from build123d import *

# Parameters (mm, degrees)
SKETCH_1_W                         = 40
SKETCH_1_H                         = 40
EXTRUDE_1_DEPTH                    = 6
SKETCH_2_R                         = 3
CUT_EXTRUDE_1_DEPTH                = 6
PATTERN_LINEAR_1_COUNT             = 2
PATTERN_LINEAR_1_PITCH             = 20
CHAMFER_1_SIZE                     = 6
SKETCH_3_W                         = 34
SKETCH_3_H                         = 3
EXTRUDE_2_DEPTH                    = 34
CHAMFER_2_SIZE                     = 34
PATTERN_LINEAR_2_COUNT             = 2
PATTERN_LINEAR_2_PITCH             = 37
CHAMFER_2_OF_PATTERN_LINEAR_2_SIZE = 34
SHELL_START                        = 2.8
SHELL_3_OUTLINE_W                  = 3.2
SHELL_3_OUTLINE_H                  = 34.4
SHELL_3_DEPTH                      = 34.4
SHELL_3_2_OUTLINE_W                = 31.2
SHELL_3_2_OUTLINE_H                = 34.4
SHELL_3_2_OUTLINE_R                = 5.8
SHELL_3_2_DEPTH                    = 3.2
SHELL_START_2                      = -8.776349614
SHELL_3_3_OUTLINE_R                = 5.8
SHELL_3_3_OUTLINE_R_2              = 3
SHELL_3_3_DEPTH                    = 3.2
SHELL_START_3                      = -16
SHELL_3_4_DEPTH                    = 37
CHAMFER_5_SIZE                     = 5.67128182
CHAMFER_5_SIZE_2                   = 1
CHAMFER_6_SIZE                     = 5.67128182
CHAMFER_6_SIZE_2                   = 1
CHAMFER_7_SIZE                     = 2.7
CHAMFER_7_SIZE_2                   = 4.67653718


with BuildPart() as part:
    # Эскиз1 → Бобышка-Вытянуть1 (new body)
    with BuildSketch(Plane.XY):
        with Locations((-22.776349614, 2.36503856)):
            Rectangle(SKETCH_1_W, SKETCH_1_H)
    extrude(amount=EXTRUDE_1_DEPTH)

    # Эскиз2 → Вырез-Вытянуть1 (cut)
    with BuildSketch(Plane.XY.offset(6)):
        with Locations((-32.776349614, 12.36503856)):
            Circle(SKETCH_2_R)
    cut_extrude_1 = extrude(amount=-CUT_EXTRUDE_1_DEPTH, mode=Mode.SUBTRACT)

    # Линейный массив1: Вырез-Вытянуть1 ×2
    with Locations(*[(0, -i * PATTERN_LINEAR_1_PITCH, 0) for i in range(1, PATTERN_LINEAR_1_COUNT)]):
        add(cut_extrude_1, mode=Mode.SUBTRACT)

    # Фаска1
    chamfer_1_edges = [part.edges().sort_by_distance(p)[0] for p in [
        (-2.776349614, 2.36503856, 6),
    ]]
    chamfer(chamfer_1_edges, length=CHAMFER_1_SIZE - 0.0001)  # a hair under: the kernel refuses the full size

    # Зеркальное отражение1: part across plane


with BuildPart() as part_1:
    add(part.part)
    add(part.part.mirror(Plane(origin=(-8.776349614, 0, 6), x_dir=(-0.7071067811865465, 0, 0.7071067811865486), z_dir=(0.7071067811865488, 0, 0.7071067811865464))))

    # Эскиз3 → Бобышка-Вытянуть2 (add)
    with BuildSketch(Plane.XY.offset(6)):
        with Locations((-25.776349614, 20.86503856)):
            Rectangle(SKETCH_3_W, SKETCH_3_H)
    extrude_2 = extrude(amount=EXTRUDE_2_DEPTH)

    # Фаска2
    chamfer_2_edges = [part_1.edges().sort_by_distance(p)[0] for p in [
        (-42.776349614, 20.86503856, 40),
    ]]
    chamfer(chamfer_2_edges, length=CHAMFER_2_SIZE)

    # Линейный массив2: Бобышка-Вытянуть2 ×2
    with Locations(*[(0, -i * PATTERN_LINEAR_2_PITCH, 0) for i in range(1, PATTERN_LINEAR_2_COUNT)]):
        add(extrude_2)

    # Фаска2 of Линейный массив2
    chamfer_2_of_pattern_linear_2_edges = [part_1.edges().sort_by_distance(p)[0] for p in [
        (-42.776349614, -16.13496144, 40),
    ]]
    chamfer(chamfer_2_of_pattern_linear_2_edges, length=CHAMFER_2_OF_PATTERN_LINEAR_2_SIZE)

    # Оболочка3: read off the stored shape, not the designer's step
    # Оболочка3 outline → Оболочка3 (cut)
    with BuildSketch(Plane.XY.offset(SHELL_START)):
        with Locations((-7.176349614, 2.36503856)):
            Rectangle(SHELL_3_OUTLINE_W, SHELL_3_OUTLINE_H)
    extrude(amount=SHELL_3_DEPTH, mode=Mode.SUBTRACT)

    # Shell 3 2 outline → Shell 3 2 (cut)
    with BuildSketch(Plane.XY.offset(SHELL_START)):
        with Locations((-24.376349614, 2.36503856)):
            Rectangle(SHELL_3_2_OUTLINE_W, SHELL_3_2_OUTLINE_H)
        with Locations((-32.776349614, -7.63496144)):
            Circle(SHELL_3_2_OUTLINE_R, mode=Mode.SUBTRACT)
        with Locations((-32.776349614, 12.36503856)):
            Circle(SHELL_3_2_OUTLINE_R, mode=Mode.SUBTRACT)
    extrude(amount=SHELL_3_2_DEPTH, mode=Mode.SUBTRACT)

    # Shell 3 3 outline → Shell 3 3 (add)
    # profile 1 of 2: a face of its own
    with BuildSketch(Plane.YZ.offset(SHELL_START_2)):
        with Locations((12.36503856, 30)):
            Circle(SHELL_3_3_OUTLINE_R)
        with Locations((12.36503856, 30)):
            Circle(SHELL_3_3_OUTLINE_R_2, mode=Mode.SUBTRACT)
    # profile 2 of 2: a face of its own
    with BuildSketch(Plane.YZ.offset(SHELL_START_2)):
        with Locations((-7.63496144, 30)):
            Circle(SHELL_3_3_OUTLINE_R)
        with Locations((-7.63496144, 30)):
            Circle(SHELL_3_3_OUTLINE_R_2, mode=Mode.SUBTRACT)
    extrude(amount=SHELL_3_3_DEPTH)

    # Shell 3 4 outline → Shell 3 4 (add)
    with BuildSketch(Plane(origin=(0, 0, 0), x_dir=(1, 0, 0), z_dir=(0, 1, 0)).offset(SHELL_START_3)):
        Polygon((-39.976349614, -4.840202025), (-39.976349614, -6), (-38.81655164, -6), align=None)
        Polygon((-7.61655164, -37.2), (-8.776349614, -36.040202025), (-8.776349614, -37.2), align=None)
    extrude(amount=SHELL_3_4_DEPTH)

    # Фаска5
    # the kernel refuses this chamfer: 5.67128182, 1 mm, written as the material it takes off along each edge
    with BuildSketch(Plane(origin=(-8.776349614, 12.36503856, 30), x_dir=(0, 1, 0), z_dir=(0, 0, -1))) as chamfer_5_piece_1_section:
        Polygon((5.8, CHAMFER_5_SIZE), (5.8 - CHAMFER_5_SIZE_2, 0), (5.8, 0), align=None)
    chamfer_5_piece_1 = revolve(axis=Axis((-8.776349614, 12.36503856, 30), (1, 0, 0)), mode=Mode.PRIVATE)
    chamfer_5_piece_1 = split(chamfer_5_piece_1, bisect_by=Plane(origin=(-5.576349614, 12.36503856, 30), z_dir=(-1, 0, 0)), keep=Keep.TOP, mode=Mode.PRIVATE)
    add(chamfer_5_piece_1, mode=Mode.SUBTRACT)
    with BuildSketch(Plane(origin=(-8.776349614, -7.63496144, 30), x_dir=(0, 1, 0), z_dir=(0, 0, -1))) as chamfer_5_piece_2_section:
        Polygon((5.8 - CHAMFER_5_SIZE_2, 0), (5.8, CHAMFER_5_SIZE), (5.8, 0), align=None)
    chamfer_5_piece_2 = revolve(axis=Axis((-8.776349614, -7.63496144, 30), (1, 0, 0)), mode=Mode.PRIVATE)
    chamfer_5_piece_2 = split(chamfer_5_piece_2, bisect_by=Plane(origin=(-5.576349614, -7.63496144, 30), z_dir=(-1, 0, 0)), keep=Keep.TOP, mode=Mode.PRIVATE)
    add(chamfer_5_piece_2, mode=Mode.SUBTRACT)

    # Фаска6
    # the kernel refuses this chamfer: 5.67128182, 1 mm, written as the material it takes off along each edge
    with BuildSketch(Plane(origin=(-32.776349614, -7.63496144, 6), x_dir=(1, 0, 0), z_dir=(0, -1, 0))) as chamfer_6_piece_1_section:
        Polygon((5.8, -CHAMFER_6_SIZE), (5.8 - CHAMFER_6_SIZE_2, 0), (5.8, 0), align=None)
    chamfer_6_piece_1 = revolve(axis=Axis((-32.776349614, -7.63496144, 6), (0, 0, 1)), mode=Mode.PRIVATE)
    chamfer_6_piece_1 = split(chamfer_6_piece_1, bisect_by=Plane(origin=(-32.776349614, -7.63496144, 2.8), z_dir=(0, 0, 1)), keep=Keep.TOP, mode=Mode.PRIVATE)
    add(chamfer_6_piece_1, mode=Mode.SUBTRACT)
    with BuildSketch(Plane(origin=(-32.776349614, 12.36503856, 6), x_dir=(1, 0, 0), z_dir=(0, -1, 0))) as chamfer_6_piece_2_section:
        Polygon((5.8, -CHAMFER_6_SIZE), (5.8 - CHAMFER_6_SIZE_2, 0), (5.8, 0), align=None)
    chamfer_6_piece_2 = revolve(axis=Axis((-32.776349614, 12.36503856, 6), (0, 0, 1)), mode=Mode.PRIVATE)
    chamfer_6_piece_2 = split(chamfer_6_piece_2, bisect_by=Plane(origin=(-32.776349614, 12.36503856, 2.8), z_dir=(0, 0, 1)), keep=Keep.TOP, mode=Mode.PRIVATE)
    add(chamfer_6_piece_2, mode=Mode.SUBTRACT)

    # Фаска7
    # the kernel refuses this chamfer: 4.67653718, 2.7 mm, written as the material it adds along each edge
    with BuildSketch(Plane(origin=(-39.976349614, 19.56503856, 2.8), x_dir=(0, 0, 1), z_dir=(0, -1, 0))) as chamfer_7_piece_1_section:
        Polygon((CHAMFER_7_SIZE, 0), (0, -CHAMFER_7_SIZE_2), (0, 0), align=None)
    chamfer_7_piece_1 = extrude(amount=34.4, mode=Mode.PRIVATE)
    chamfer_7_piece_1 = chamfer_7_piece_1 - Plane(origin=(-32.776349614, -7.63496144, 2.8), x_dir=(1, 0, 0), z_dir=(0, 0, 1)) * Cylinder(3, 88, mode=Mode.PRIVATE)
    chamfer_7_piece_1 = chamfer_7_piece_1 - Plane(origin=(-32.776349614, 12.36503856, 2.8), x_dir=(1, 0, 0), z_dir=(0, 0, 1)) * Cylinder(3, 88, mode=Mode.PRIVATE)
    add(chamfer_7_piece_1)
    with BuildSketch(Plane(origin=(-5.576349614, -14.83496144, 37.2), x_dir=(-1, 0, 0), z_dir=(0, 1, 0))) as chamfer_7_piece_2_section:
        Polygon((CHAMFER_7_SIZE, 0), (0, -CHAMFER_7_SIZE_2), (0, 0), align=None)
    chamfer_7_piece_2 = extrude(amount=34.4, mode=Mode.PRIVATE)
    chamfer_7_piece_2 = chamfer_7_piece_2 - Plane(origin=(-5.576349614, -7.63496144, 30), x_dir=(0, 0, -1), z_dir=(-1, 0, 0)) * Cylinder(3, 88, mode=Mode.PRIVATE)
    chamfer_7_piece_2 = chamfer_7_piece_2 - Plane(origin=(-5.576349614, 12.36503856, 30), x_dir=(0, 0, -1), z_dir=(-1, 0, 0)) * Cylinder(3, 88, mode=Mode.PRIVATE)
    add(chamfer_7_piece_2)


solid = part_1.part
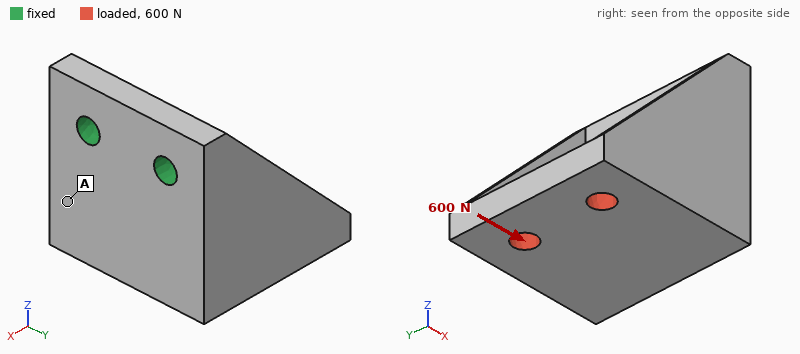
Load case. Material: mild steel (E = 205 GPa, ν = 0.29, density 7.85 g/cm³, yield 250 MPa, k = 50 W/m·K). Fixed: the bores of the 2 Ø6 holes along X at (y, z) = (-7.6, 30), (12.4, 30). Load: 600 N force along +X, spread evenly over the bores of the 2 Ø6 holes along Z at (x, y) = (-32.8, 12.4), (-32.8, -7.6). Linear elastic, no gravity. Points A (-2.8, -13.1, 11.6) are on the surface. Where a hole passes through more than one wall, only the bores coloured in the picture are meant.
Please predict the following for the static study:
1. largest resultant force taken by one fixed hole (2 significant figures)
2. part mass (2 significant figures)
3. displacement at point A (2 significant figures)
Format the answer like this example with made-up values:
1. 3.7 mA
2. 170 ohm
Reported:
1. 310 N
2. 120 g
3. 25 µm
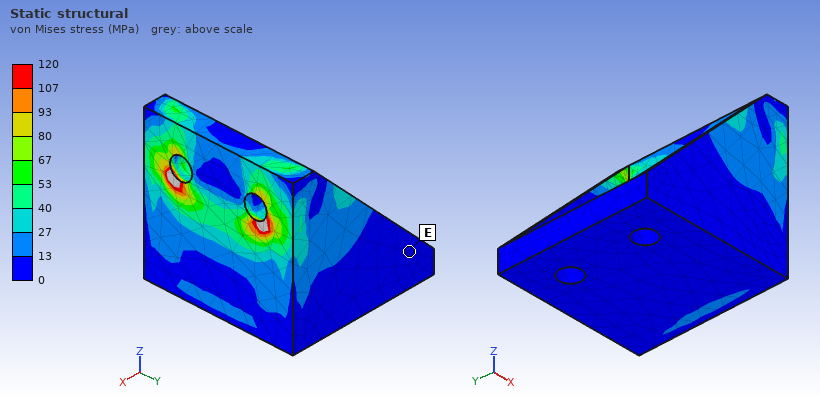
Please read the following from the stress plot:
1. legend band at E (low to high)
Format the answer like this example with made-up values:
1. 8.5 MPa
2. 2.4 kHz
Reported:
1. 0 to 13 MPa
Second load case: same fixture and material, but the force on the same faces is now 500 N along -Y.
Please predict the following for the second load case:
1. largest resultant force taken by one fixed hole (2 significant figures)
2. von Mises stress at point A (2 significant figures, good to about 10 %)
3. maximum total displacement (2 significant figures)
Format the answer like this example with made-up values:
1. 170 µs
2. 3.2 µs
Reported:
1. 670 N
2. 18 MPa
3. 0.10 mm
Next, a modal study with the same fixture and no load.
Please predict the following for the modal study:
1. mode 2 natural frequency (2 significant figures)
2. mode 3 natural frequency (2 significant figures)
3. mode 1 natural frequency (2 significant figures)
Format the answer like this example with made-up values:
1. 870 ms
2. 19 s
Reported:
1. 1900 Hz
2. 6800 Hz
3. 1900 Hz
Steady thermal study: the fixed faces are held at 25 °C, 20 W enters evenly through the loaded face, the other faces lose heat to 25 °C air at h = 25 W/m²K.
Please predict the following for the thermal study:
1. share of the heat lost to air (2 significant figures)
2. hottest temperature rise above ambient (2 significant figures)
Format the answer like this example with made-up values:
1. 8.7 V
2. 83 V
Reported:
1. 42 %
2. 76 K
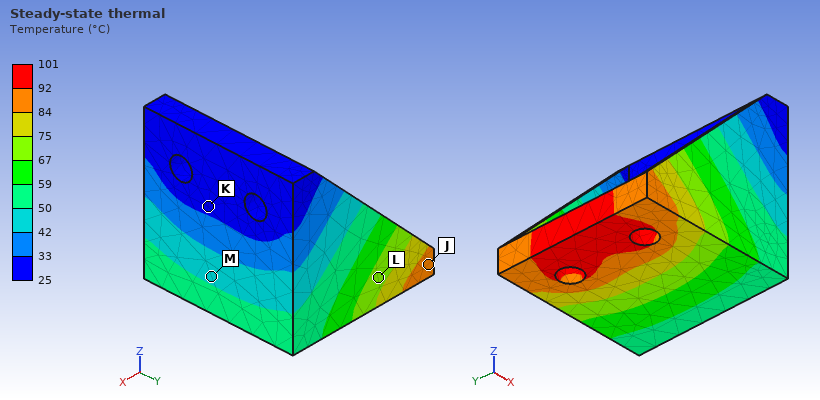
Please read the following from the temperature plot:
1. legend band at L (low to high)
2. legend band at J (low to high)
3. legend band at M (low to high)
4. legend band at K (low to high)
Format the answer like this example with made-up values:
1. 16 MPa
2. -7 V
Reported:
1. 67 to 75 °C
2. 84 to 92 °C
3. 42 to 50 °C
4. 25 to 33 °C
